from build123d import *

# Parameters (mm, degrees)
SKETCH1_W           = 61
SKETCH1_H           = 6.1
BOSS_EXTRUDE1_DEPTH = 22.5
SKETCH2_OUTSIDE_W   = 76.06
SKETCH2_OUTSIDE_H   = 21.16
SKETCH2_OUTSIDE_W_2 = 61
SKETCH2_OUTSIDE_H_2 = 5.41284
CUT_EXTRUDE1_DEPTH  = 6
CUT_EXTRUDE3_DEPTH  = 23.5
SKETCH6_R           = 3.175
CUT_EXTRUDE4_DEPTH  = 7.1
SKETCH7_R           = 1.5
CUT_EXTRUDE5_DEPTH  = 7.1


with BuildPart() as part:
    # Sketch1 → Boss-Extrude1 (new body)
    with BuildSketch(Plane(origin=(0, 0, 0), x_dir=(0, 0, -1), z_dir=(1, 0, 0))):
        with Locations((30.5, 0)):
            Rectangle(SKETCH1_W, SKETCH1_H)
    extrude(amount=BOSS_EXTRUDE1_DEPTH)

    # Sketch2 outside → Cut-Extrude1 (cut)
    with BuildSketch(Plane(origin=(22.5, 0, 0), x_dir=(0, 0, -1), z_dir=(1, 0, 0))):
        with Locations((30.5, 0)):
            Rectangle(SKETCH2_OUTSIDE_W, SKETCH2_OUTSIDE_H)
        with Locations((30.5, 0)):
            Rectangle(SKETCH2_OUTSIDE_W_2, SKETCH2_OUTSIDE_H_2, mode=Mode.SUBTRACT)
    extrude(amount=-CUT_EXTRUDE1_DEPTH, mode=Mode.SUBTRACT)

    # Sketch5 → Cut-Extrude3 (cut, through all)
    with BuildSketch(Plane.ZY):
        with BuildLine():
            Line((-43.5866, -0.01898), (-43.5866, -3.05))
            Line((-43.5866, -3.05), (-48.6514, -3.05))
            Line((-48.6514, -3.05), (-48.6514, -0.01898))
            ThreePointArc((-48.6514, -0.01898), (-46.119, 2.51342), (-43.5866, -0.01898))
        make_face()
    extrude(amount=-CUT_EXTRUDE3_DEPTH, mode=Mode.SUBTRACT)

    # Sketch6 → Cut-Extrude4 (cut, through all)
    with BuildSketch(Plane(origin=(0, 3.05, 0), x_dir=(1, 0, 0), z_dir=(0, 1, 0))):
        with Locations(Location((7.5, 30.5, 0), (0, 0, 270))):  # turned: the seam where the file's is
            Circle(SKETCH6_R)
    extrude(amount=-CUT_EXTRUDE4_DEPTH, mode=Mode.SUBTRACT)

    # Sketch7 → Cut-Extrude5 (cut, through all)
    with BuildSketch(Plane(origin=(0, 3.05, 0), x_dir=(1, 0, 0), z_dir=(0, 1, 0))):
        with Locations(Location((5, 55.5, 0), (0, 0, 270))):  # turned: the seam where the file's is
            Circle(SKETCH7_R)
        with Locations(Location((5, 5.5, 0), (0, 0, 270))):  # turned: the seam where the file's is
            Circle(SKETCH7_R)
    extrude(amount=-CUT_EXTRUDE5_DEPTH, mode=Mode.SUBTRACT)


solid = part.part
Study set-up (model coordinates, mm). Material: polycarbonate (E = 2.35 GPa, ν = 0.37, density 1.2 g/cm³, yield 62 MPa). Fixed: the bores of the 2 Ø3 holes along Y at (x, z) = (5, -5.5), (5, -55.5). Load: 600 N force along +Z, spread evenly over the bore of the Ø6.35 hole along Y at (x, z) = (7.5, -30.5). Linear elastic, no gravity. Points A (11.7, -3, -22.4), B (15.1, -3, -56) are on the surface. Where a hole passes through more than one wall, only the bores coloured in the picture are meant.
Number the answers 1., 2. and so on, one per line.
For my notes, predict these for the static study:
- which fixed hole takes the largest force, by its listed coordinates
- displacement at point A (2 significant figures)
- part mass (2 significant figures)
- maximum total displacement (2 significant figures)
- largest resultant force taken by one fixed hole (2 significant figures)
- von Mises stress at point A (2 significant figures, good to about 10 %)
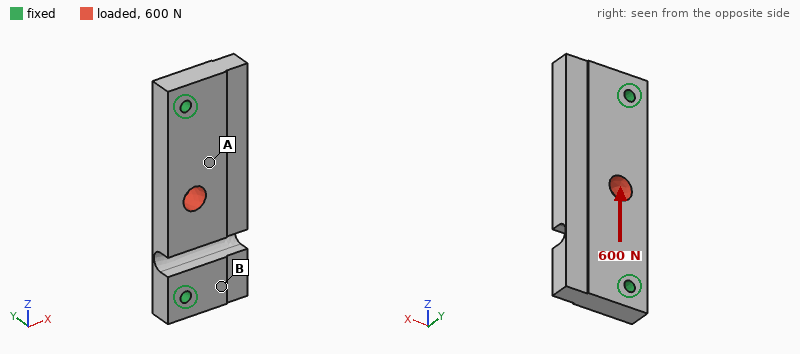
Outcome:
1. (5, -5.5)
2. 0.064 mm
3. 8.7 g
4. 0.11 mm
5. 470 N
6. 5.1 MPa
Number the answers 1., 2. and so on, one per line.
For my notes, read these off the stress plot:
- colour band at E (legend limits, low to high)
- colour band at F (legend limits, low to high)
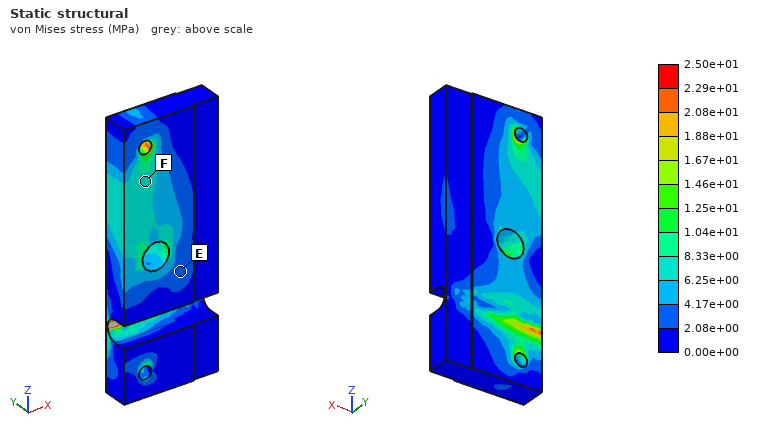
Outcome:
1. 2.08e+00 to 4.17e+00 MPa
2. 6.25e+00 to 8.33e+00 MPa
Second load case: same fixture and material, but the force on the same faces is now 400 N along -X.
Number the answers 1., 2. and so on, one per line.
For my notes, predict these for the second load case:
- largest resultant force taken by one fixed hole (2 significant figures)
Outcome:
1. 230 N
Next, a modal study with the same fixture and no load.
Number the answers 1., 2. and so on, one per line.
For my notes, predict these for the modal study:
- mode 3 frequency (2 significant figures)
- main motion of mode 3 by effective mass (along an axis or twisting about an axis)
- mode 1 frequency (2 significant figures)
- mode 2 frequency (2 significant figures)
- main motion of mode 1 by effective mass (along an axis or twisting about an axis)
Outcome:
1. 3700 Hz
2. along X
3. 1800 Hz
4. 2600 Hz
5. along Y
